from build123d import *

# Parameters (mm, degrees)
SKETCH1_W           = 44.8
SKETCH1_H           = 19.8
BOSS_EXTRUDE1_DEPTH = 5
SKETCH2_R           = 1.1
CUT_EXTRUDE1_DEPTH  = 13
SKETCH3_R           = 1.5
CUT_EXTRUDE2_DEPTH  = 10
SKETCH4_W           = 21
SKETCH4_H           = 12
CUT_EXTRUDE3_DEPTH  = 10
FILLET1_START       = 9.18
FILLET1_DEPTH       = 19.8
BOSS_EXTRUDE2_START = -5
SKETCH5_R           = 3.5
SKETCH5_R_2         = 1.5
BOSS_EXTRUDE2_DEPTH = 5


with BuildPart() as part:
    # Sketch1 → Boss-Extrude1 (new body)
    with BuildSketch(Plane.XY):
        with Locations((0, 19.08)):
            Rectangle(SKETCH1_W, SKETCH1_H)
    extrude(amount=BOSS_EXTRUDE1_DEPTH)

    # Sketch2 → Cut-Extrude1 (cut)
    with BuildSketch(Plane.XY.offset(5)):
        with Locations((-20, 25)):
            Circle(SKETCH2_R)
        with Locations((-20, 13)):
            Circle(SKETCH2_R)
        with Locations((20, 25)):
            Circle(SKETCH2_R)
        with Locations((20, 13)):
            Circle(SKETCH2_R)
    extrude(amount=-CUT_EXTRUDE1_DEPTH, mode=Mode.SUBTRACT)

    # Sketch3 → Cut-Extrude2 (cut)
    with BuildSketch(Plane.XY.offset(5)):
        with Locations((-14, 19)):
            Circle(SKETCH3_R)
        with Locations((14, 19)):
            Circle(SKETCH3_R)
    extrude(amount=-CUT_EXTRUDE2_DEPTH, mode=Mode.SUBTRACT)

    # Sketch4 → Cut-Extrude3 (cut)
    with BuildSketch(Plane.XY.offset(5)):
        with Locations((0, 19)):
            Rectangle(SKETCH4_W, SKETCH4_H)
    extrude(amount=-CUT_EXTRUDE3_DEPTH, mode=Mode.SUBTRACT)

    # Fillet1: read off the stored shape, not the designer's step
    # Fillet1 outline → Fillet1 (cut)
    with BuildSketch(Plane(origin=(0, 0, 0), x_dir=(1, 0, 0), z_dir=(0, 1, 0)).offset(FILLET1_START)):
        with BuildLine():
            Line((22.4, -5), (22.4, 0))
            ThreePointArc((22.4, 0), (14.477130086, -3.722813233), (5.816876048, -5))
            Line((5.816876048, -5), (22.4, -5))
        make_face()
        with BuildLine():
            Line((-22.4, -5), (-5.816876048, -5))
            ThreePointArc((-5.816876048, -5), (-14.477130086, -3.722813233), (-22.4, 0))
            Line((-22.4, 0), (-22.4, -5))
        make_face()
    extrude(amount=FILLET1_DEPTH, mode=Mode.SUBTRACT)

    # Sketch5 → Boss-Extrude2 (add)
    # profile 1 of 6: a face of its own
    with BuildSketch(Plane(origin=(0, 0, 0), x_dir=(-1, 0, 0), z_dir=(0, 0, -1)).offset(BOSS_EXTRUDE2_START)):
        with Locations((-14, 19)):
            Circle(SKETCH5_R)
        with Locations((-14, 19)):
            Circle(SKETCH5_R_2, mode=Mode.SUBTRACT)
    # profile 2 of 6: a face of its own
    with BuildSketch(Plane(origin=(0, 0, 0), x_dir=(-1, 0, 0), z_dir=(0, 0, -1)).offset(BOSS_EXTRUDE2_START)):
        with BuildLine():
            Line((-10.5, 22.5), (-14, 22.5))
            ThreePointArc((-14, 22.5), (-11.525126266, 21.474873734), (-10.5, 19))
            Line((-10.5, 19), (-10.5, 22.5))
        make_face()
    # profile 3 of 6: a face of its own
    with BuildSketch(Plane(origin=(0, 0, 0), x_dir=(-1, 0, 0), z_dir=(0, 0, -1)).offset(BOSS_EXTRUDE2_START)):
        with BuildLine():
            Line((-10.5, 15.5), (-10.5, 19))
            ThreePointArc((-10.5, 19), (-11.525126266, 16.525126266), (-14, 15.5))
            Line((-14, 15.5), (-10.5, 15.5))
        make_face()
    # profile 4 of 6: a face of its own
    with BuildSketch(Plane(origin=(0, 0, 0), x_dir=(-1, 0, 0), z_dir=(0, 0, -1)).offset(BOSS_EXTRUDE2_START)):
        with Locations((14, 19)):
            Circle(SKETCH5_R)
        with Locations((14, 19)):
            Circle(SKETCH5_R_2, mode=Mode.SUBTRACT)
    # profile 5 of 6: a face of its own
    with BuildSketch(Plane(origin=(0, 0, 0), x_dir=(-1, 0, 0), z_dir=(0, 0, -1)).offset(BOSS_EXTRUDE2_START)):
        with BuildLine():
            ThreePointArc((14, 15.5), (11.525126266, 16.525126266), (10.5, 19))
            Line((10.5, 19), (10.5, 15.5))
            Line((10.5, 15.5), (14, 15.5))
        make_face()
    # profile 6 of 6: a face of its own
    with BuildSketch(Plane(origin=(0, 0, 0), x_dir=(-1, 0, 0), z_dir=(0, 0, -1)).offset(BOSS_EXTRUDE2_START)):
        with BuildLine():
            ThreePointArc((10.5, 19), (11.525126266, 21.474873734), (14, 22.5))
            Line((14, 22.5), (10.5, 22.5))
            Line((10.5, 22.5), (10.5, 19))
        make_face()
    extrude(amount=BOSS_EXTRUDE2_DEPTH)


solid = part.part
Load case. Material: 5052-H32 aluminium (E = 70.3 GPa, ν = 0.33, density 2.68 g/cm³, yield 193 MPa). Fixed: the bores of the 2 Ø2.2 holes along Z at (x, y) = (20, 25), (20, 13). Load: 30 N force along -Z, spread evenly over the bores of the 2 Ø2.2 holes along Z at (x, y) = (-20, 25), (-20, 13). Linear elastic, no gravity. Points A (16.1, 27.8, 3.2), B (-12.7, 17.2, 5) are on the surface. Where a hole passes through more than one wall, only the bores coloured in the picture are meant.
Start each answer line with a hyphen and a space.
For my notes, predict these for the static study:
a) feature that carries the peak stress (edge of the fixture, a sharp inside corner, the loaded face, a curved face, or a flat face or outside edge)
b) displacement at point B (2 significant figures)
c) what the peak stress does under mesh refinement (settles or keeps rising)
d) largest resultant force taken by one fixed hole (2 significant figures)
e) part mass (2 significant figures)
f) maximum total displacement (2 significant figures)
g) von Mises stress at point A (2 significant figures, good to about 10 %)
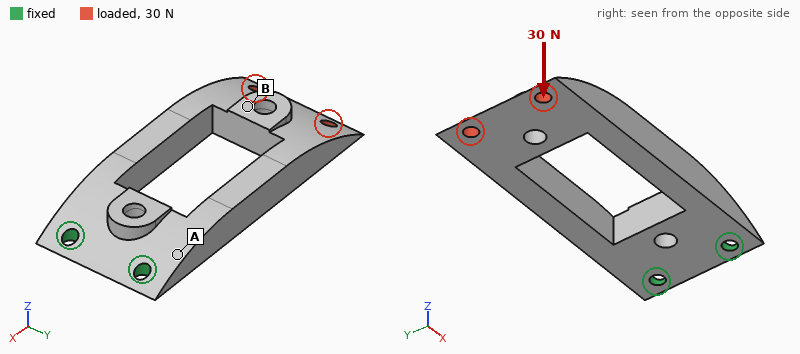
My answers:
- edge of the fixture
- 0.20 mm
- keeps rising
- 15 N
- 5.7 g
- 0.28 mm
- 37 MPa
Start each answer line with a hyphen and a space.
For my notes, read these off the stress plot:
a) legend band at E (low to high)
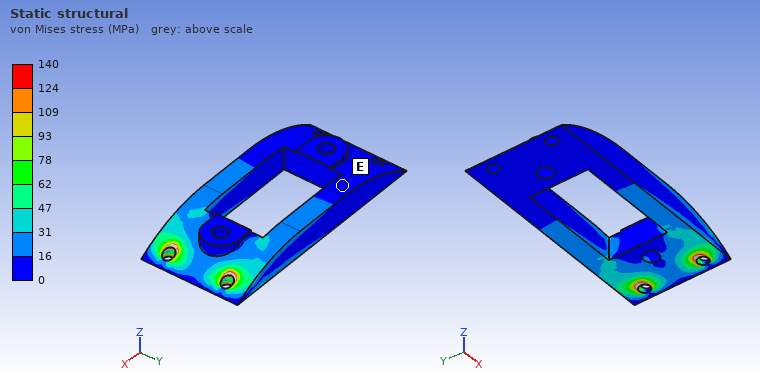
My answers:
- 0 to 16 MPa
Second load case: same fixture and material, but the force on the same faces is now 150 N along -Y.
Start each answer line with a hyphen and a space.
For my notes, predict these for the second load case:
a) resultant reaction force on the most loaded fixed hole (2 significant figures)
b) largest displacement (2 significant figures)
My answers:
- 450 N
- 0.13 mm
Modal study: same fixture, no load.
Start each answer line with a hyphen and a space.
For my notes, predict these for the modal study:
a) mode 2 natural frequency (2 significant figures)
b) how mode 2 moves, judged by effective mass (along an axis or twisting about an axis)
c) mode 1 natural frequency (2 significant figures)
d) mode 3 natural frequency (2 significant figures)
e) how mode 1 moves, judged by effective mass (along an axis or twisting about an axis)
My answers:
- 3900 Hz
- along Y
- 1300 Hz
- 5500 Hz
- along Z
